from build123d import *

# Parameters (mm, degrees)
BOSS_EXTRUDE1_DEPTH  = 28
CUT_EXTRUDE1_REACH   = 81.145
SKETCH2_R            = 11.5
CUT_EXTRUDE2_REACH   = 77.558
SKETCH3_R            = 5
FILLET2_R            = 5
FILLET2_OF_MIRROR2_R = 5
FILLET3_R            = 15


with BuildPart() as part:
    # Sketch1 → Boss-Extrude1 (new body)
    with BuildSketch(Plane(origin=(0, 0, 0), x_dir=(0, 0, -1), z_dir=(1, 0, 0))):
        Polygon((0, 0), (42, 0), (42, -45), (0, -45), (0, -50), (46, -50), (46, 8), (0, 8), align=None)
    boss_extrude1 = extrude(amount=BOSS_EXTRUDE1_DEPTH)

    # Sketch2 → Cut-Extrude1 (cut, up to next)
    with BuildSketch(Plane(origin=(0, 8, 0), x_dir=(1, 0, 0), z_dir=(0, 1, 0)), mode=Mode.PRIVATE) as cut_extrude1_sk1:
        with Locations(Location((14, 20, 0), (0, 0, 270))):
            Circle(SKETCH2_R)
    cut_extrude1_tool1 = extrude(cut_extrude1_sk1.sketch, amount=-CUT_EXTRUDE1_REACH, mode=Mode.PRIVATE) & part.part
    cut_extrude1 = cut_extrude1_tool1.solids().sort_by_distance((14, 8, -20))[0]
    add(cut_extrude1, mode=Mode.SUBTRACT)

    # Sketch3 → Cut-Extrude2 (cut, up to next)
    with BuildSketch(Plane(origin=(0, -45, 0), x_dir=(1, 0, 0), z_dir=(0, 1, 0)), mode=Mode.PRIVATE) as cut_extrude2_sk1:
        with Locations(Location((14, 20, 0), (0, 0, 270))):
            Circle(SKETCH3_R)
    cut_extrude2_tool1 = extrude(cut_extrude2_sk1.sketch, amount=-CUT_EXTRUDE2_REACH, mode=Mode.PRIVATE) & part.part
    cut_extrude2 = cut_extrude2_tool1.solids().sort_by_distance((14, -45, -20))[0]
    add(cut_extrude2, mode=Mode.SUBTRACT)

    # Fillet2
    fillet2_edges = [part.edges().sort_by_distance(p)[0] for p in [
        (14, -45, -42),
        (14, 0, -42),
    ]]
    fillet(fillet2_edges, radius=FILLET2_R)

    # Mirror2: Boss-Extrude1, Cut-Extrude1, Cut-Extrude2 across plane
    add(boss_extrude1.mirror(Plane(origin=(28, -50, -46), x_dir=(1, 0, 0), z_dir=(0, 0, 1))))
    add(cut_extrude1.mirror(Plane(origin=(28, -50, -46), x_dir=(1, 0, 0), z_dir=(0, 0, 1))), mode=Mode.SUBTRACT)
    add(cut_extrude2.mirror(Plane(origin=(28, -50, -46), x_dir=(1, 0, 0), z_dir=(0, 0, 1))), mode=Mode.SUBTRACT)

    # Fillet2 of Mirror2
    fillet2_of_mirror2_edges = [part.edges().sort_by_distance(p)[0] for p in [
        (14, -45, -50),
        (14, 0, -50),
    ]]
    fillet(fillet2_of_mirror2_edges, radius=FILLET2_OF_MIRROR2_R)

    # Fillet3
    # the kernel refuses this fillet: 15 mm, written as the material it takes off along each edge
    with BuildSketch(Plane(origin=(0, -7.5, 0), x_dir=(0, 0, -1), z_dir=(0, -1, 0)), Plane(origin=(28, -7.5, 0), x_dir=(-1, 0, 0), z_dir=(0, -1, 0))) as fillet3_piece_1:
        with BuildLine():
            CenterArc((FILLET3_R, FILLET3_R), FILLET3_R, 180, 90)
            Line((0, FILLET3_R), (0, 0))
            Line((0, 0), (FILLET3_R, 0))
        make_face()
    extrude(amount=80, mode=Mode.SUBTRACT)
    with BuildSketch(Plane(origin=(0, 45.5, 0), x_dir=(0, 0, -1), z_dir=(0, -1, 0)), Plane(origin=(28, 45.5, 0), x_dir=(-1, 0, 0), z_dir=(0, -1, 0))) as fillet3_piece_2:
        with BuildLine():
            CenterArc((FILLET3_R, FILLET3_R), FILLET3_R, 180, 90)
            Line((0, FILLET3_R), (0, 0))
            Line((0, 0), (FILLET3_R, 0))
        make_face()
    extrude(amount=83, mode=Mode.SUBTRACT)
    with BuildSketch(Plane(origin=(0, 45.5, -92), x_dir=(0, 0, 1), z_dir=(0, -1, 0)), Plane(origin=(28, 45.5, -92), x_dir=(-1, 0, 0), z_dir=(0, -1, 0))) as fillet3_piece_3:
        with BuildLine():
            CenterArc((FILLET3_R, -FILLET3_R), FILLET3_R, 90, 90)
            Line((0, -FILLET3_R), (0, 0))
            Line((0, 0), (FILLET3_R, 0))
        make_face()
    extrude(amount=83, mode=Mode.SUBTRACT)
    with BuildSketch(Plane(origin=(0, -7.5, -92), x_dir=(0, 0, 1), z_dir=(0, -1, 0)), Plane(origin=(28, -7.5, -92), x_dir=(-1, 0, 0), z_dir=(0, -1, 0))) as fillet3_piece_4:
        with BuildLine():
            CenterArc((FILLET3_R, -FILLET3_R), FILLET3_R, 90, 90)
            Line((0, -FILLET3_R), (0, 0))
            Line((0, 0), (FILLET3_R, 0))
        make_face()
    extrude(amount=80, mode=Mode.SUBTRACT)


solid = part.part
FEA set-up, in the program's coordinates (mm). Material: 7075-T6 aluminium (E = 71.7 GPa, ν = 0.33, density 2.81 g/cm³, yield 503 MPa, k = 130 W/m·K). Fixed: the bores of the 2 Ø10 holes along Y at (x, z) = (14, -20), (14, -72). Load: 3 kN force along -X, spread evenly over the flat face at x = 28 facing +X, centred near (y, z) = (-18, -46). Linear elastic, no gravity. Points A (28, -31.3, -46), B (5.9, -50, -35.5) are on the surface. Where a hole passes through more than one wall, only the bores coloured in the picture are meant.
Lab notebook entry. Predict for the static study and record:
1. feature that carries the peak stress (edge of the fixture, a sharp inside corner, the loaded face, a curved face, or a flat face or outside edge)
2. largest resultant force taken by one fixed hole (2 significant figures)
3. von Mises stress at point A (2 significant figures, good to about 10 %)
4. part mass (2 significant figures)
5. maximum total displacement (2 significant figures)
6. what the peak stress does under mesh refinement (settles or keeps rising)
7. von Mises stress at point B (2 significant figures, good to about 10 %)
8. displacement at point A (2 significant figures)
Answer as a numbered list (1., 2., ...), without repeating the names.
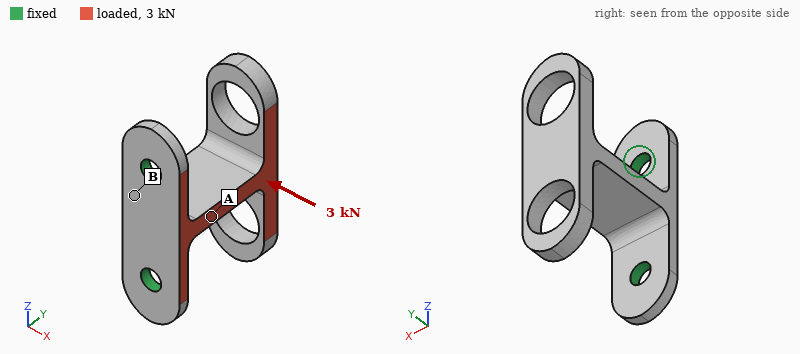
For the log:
1. edge of the fixture
2. 1.5 kN
3. 54 MPa
4. 96 g
5. 1.1 mm
6. keeps rising
7. 180 MPa
8. 0.41 mm
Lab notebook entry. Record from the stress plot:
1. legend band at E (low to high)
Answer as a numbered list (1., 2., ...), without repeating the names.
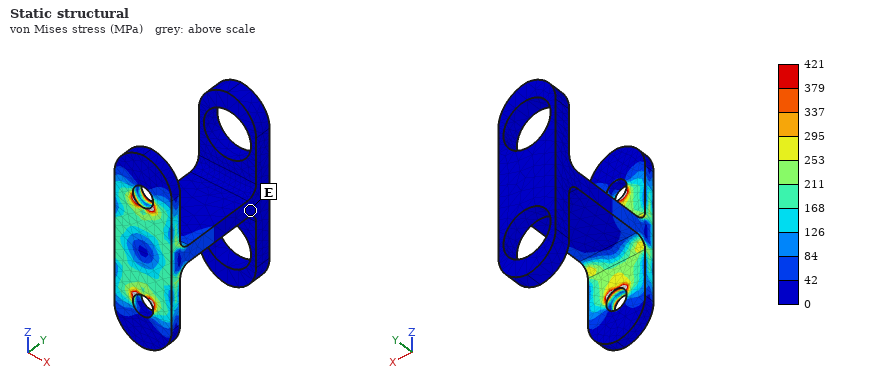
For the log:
1. 0 to 42 MPa
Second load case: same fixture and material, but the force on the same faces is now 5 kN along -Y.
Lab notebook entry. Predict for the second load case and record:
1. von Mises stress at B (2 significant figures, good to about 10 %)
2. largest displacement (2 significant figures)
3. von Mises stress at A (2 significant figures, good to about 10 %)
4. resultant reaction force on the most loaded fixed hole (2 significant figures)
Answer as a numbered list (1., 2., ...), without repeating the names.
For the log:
1. 120 MPa
2. 0.83 mm
3. 56 MPa
4. 2.7 kN
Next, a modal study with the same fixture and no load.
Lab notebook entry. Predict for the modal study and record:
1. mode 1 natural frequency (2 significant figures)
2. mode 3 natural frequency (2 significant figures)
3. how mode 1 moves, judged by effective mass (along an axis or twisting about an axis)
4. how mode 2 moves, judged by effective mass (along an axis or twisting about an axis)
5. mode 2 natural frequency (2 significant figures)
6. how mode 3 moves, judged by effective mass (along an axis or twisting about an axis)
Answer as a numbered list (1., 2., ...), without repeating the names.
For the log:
1. 850 Hz
2. 1700 Hz
3. along Z
4. along X
5. 970 Hz
6. twisting about Y
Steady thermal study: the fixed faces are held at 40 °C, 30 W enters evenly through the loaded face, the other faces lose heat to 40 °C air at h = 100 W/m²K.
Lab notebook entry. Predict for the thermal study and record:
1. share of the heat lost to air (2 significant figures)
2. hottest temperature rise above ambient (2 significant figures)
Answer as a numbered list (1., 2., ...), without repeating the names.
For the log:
1. 45 %
2. 21 K
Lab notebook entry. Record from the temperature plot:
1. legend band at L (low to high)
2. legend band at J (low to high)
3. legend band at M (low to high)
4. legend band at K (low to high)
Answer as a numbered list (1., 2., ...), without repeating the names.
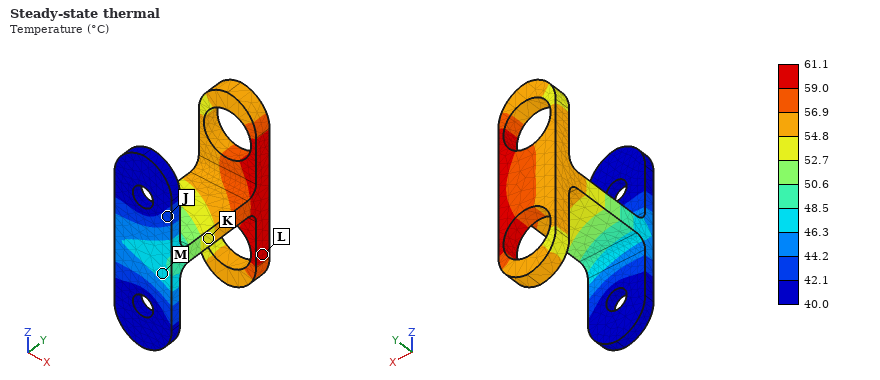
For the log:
1. 59.0 to 61.1 °C
2. 42.1 to 44.2 °C
3. 46.3 to 48.5 °C
4. 52.7 to 54.8 °C
